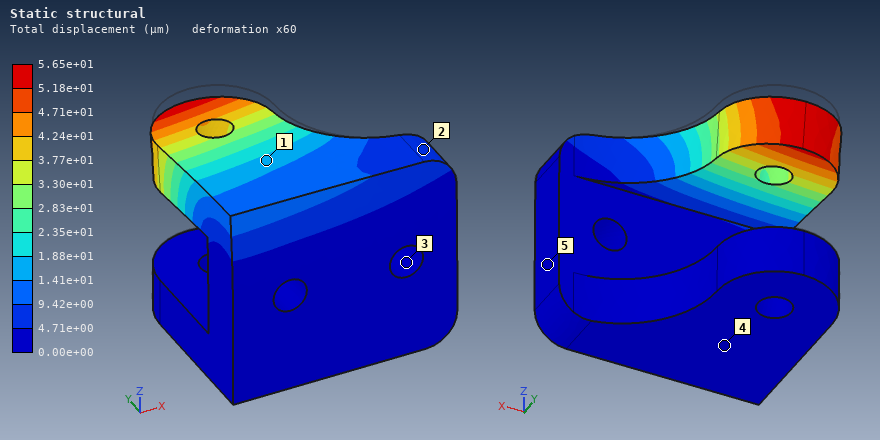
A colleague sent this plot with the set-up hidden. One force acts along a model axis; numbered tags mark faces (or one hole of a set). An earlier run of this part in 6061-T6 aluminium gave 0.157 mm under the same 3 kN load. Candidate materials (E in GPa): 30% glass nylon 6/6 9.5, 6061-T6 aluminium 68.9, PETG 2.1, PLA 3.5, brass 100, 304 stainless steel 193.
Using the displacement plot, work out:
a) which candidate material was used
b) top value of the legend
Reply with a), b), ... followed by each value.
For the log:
a) 304 stainless steel
b) 5.65e+01 µm
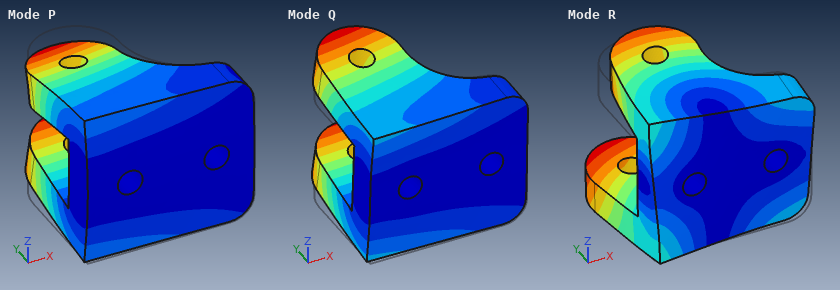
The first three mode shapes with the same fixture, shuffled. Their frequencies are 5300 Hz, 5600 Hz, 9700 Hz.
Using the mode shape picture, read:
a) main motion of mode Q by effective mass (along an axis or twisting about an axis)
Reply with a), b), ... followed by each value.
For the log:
a) along Z
